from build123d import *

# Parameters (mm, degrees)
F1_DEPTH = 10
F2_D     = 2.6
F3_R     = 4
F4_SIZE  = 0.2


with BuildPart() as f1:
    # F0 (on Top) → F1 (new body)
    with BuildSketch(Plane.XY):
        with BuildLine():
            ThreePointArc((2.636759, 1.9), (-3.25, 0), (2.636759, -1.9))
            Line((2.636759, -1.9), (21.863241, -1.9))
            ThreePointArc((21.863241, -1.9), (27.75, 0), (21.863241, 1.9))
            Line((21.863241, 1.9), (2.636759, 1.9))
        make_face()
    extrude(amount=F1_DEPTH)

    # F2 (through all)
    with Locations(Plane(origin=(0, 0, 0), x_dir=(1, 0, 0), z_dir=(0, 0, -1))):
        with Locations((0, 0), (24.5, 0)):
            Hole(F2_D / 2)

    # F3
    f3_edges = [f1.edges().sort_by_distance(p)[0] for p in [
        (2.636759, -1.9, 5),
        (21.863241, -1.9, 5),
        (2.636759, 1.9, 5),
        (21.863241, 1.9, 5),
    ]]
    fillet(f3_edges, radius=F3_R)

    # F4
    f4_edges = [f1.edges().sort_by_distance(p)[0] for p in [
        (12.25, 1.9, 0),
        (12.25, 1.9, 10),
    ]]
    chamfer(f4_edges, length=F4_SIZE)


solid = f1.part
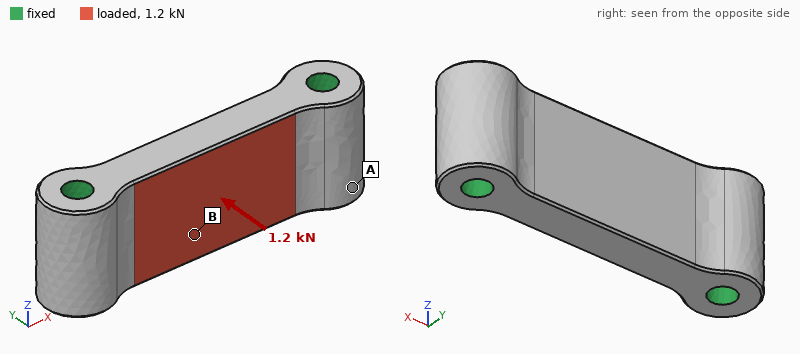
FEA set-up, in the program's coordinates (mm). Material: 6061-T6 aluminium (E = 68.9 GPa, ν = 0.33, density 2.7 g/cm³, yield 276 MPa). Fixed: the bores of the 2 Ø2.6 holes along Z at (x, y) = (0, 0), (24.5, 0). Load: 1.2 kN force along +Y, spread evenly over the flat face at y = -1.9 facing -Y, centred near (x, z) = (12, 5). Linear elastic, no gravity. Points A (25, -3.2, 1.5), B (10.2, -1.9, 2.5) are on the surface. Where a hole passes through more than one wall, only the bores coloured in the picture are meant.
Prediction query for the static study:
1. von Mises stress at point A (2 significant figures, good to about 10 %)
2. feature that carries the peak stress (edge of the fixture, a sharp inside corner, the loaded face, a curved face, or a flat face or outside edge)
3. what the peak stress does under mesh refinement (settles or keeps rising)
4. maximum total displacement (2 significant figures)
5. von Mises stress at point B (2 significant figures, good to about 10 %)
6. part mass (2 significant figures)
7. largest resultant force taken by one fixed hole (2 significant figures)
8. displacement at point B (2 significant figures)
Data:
12 MPa
edge of the fixture
keeps rising
19 µm
49 MPa
3.4 g
600 N
17 µm
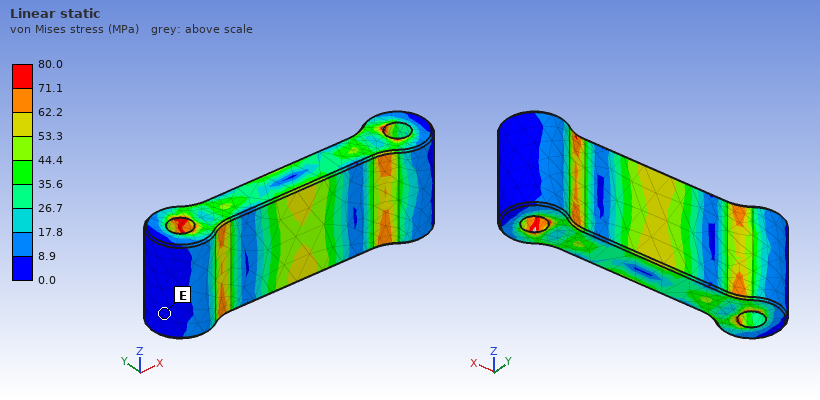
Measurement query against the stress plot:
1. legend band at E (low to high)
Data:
0.0 to 8.9 MPa
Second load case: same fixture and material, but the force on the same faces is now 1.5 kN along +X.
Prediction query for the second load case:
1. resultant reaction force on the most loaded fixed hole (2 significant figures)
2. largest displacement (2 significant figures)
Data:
760 N
2.8 µm
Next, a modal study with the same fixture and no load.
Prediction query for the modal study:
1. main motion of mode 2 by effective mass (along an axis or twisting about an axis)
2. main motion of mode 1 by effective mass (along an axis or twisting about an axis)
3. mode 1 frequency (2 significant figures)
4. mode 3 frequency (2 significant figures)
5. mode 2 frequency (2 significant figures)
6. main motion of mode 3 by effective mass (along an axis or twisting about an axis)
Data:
twisting about X
along Y
35 kHz
56 kHz
53 kHz
along Z
